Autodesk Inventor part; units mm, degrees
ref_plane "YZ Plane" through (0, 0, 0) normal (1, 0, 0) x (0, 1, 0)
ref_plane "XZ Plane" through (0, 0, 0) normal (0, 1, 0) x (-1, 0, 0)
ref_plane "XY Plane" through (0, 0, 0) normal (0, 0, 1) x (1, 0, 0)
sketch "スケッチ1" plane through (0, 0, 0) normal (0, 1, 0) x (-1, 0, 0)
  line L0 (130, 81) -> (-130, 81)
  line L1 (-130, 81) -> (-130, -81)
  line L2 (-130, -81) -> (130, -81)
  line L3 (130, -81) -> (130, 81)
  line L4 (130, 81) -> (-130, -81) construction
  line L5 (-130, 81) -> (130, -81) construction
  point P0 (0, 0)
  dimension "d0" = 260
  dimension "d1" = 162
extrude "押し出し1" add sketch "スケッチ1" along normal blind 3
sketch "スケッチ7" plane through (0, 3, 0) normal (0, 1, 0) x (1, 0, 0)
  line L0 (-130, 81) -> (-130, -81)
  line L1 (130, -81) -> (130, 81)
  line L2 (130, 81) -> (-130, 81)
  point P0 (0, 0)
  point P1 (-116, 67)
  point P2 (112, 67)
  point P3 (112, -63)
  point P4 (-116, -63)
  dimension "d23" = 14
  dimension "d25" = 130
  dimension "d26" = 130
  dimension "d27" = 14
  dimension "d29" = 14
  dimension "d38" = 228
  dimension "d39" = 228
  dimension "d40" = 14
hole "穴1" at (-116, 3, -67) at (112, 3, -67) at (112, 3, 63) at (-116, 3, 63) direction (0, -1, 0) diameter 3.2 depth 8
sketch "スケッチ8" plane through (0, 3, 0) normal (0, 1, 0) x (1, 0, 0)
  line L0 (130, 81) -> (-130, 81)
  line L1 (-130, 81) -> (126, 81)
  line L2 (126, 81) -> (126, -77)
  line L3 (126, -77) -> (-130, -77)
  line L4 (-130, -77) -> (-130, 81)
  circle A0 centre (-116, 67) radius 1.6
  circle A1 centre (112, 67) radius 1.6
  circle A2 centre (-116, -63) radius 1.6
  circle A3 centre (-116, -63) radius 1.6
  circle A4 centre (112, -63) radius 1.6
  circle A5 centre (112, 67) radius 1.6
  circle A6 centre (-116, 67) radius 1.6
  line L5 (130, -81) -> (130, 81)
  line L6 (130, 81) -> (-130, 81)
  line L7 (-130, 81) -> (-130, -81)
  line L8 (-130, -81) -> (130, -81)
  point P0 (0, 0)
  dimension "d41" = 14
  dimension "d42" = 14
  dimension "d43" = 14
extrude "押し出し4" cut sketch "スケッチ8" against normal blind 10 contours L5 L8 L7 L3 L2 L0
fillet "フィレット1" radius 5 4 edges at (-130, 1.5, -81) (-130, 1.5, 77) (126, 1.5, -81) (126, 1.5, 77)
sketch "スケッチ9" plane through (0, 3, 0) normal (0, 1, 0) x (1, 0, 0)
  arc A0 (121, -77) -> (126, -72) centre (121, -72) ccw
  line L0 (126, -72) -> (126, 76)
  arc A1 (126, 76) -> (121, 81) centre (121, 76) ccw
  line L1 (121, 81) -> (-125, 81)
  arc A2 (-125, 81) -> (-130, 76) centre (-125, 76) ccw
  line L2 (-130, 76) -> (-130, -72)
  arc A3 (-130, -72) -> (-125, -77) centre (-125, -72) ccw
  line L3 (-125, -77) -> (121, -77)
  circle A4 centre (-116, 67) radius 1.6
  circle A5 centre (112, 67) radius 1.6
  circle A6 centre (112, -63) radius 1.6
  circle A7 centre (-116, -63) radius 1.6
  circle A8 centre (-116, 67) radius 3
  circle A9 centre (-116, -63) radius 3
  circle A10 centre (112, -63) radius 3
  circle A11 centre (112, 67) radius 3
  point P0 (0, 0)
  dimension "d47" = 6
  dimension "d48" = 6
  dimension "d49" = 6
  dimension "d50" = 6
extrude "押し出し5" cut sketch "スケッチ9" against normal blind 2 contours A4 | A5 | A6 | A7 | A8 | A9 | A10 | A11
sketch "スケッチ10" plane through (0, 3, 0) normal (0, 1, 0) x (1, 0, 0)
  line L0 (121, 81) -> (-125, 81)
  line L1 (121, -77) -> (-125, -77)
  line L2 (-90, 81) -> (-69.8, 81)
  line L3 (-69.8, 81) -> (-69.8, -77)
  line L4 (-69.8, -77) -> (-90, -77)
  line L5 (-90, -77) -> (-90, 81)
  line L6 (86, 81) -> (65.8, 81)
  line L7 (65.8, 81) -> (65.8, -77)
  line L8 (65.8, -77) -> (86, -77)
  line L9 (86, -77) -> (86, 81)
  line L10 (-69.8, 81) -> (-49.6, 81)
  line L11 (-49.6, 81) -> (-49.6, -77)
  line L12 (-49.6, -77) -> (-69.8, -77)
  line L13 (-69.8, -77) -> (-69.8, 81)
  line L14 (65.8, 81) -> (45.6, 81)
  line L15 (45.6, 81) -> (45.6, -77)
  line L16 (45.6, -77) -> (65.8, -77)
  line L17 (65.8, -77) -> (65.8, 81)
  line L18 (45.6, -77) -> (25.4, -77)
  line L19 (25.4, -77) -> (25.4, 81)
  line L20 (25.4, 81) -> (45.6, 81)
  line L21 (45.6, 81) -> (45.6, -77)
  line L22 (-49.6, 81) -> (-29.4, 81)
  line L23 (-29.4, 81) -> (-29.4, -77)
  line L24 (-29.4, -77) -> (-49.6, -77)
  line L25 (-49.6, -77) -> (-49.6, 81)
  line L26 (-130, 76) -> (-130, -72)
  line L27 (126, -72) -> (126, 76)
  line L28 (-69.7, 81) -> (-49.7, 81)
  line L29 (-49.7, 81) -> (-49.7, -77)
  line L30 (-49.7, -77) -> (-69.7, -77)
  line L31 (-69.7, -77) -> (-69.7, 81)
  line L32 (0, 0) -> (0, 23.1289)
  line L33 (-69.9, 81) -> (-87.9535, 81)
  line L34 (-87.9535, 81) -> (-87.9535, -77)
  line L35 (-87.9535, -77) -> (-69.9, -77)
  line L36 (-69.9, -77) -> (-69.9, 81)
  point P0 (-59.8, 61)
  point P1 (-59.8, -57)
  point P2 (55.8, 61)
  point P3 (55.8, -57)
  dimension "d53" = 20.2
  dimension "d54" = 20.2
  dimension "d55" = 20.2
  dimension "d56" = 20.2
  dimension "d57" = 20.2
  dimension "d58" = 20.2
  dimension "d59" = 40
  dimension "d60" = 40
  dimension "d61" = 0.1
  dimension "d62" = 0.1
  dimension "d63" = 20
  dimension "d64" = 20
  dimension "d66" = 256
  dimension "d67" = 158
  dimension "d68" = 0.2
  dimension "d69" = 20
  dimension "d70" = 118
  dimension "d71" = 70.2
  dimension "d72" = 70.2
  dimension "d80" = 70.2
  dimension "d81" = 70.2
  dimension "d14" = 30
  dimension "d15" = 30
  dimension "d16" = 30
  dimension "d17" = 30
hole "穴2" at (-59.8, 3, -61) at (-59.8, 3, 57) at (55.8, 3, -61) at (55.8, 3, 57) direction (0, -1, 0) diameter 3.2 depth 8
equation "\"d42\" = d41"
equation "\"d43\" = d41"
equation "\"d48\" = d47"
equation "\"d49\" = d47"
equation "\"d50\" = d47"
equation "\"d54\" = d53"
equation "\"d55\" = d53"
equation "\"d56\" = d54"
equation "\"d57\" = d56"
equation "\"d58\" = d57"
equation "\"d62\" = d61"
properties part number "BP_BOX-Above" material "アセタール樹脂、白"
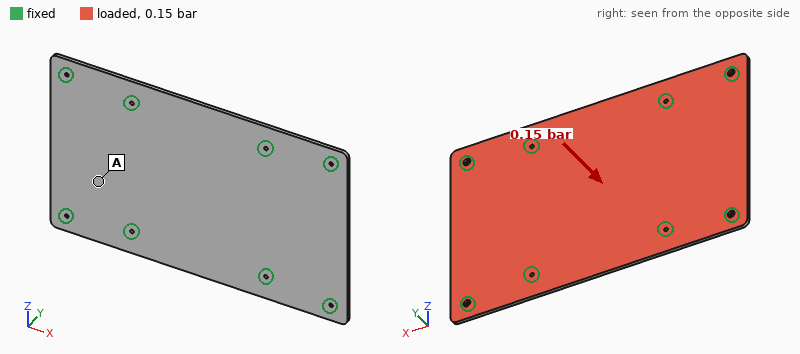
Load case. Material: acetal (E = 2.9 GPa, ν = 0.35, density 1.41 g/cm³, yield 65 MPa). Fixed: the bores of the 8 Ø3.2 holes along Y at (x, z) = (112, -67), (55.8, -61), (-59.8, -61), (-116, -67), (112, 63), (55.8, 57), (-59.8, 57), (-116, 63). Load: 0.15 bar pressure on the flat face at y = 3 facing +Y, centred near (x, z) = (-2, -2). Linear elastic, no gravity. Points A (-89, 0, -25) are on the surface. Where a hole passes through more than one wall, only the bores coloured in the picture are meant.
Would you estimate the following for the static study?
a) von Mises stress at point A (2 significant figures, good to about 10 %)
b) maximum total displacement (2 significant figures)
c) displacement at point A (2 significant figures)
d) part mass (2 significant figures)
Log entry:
4.5 MPa
2.9 mm
1.7 mm
170 g
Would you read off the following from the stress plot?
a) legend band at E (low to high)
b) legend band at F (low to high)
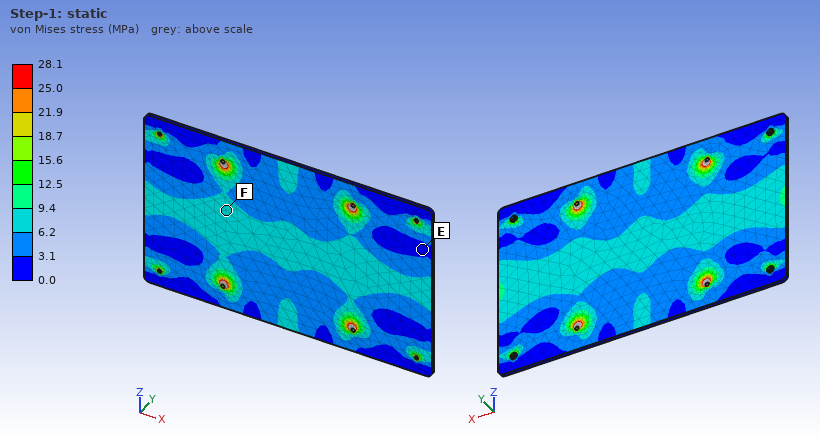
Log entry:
0.0 to 3.1 MPa
6.2 to 9.4 MPa
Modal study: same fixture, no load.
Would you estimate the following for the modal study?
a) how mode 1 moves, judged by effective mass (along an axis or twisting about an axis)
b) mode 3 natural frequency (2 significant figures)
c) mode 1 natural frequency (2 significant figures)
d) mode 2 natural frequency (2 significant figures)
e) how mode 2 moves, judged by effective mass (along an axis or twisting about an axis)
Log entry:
along Y
240 Hz
210 Hz
230 Hz
twisting about Z
